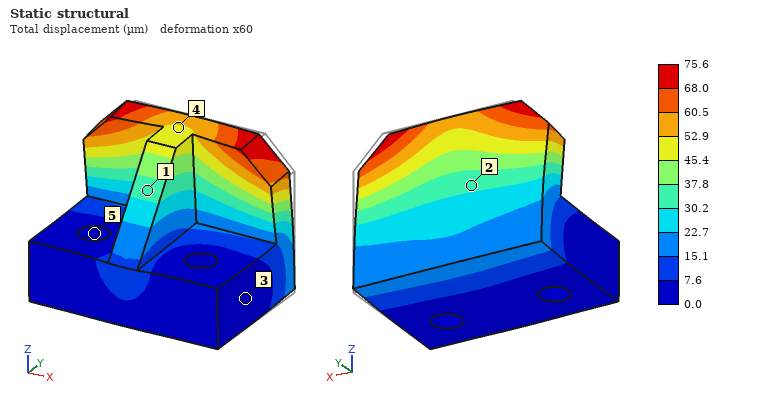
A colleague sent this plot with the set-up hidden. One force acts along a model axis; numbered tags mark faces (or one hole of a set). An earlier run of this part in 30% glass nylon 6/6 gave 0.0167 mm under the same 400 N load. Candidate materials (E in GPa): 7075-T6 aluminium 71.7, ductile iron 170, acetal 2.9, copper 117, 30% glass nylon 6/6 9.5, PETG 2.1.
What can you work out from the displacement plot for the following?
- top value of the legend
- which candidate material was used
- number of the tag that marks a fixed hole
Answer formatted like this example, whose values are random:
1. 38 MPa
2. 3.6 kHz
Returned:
1. 75.6 µm
2. PETG
3. 5
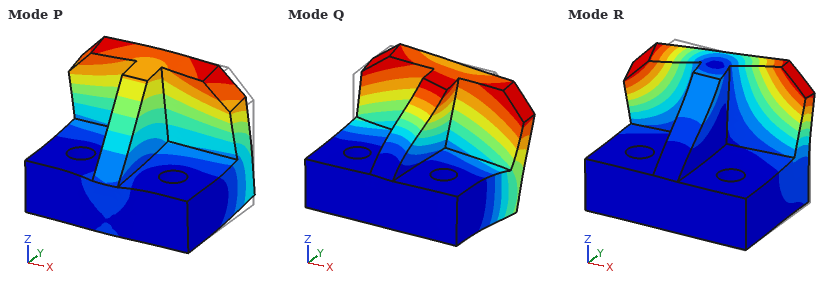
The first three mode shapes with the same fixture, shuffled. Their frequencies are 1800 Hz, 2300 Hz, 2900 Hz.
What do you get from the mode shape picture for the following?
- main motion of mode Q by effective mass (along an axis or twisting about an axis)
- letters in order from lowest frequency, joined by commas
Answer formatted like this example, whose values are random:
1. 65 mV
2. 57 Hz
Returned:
1. along X
2. P, Q, R
